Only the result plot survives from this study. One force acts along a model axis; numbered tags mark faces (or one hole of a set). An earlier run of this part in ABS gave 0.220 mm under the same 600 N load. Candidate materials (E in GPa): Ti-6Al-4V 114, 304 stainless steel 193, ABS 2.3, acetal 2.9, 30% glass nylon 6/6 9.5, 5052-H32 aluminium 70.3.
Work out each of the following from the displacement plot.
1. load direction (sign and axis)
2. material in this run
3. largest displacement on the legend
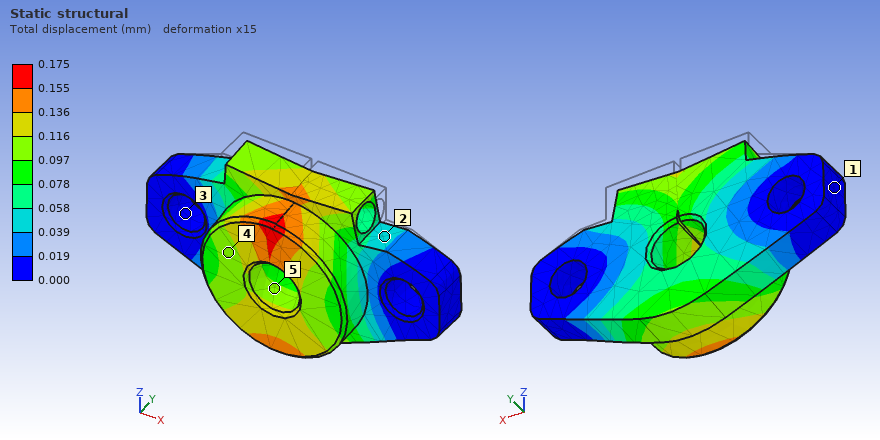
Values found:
-Z
acetal
0.175 mm
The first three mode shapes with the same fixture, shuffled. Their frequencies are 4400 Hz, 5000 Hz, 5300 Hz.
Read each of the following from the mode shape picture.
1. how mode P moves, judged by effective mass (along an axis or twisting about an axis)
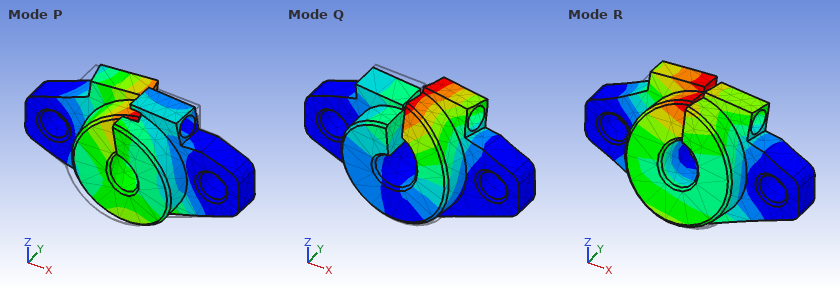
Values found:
along Y
